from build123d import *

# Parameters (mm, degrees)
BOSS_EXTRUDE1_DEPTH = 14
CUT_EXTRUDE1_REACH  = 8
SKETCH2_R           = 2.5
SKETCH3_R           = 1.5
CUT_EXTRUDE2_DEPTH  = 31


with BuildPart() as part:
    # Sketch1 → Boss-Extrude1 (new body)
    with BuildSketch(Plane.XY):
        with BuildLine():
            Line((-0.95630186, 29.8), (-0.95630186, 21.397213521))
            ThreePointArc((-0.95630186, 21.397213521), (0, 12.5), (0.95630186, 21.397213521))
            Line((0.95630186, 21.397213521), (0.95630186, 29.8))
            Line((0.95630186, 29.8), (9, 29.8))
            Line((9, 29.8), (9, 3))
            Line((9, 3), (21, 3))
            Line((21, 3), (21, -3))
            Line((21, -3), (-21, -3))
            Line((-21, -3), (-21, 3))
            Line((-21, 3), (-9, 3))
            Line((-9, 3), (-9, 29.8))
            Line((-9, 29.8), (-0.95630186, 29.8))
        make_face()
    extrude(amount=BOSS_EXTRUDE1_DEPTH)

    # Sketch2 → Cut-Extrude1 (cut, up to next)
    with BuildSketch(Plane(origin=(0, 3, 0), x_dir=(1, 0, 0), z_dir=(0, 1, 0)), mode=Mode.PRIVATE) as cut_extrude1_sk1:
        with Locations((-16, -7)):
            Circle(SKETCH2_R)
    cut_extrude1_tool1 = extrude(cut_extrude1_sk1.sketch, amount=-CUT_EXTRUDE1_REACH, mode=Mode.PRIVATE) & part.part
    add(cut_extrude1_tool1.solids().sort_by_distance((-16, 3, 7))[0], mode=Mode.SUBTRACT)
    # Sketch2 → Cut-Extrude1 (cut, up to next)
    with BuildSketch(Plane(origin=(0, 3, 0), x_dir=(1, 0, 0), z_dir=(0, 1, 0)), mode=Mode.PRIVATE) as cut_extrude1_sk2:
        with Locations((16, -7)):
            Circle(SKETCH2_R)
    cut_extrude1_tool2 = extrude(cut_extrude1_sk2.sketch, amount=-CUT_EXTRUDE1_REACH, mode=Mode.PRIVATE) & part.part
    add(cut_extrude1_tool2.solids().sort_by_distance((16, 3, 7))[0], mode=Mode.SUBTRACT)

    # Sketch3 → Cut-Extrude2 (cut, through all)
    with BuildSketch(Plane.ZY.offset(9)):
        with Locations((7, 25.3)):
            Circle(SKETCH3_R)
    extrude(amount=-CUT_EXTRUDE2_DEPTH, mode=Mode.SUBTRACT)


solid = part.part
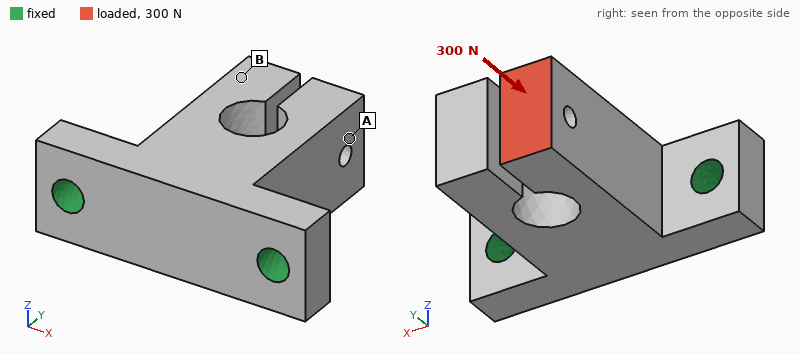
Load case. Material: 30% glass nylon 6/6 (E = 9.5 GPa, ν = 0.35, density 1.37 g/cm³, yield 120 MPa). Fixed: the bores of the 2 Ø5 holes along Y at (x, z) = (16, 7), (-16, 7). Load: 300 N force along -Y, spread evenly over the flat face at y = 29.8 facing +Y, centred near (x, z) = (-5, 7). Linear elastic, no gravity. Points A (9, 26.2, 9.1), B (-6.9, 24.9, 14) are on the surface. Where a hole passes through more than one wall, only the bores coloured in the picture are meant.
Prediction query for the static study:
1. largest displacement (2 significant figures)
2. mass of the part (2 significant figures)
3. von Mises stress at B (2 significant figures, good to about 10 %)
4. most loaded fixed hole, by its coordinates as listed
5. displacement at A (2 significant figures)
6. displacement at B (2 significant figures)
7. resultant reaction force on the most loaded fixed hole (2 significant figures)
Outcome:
48 µm
12 g
2.7 MPa
(-16, 7)
11 µm
23 µm
220 N
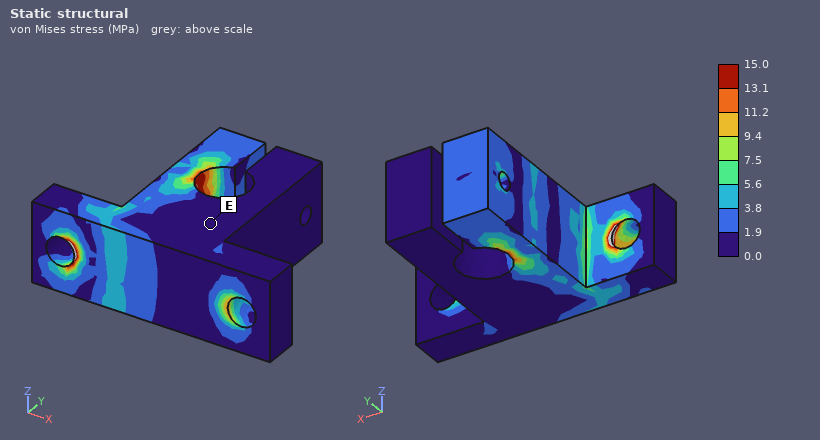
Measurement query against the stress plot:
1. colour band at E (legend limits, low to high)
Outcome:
0.0 to 1.9 MPa
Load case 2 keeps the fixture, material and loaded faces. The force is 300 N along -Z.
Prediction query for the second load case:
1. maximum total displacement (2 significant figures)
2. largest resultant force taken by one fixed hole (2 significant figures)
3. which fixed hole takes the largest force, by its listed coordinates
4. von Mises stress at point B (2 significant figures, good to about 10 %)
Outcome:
0.52 mm
190 N
(-16, 7)
7.9 MPa
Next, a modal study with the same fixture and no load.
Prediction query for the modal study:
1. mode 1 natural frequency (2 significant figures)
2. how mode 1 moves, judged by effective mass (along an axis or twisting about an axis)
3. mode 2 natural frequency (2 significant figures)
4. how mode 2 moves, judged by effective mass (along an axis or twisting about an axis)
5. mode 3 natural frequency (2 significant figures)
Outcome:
2600 Hz
along Z
3900 Hz
along X
4600 Hz
